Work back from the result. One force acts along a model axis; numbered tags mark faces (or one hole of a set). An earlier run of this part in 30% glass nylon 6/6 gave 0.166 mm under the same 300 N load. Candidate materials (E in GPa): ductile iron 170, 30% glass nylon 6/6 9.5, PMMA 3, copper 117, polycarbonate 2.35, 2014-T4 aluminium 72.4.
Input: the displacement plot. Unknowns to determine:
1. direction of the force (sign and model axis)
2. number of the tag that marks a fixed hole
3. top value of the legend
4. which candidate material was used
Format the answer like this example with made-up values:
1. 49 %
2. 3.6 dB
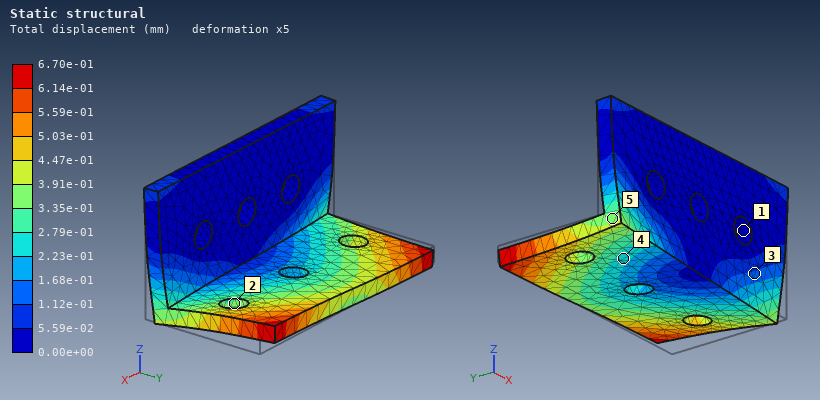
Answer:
1. -X
2. 1
3. 6.70e-01 mm
4. polycarbonate
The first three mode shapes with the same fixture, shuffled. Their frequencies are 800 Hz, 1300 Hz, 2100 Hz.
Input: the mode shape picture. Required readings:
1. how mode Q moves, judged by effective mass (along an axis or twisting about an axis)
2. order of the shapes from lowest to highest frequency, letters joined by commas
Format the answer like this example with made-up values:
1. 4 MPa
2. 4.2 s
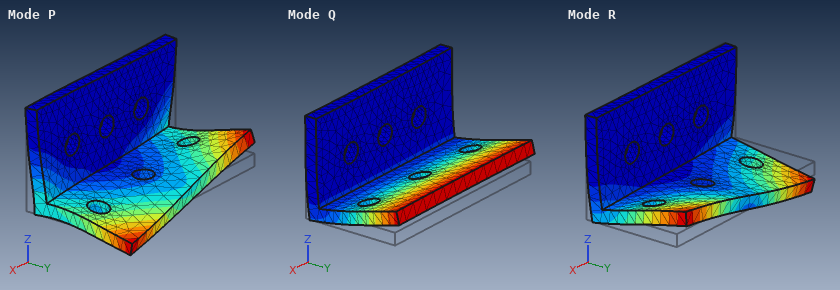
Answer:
1. along Z
2. Q, R, P
